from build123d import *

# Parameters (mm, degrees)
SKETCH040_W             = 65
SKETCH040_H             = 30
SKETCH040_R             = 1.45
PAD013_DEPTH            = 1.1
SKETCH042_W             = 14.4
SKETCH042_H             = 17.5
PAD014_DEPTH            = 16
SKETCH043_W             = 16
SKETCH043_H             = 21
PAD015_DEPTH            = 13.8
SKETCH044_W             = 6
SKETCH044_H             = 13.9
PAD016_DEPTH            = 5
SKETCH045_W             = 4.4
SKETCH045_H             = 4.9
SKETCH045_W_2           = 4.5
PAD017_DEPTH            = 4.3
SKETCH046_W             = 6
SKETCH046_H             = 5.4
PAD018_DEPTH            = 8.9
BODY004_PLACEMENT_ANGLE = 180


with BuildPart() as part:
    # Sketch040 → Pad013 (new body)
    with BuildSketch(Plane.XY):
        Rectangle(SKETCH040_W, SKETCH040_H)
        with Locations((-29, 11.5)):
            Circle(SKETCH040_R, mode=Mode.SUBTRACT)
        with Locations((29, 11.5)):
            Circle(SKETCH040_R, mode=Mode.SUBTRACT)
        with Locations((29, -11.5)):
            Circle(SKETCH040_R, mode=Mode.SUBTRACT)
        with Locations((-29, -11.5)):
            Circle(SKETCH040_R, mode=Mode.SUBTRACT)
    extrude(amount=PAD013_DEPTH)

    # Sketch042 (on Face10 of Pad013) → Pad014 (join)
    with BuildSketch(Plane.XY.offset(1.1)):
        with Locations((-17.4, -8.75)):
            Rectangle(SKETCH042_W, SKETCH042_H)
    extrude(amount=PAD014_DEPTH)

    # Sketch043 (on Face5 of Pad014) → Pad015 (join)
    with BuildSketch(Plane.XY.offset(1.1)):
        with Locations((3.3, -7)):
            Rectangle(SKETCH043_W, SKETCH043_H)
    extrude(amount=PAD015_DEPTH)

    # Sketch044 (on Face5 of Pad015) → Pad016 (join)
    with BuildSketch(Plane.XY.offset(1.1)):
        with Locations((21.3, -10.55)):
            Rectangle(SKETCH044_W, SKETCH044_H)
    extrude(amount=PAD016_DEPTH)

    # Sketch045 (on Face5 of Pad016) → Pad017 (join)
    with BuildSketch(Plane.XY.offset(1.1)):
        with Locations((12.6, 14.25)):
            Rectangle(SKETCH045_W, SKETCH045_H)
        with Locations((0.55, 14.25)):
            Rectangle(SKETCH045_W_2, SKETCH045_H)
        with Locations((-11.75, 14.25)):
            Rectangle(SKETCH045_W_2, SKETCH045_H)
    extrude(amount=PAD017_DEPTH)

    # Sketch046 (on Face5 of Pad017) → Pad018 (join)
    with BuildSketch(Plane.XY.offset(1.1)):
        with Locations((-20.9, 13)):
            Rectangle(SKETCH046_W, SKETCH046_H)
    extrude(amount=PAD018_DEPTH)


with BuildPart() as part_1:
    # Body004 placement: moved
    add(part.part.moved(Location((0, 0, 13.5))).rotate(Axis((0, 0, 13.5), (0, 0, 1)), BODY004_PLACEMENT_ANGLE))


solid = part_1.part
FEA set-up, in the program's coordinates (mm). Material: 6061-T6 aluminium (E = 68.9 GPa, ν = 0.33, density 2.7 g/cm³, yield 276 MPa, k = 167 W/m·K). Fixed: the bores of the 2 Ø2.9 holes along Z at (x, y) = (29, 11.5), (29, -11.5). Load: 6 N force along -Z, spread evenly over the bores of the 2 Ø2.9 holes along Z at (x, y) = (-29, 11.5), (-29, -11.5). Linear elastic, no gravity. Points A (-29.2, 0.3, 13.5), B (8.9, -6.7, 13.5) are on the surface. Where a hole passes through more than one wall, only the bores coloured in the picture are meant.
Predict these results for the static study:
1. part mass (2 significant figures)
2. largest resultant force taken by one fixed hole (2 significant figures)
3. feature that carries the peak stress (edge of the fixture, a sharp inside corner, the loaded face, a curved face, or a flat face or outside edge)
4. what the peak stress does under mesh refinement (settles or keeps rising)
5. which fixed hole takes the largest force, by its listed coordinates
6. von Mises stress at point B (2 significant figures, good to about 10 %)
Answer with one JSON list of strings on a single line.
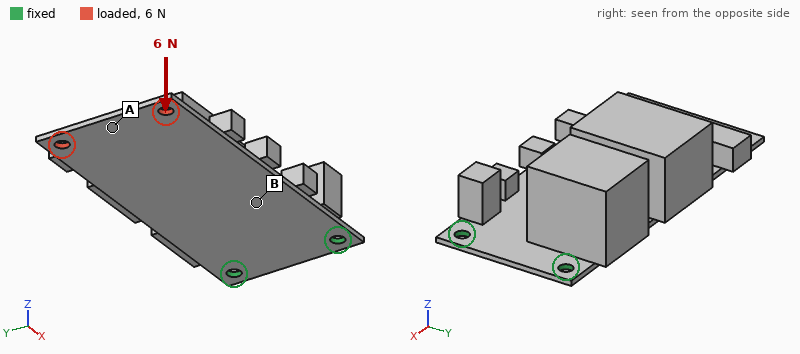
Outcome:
["32 g", "5.6 N", "edge of the fixture", "keeps rising", "(29, -11.5)", "23 MPa"]
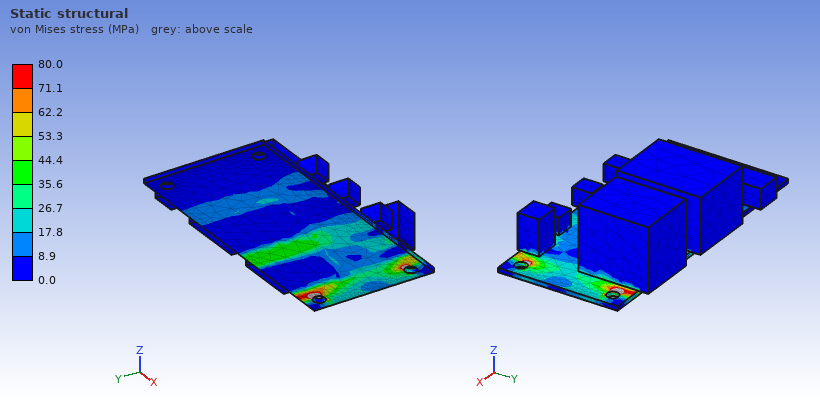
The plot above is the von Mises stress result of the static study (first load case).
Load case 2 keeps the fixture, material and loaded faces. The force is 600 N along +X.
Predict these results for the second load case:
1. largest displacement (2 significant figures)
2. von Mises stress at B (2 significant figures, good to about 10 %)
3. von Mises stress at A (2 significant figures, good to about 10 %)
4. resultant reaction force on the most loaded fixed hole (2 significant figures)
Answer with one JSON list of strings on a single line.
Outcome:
["76 µm", "17 MPa", "8.7 MPa", "310 N"]
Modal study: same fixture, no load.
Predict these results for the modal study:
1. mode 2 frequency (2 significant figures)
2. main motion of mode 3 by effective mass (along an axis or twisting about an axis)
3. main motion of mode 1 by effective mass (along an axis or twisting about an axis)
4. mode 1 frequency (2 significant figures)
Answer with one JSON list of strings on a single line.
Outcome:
["910 Hz", "along Y", "along Z", "190 Hz"]
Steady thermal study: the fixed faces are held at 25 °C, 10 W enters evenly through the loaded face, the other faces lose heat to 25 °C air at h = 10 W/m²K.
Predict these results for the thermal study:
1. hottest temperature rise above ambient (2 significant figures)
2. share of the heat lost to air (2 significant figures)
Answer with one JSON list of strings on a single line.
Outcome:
["77 K", "20 %"]
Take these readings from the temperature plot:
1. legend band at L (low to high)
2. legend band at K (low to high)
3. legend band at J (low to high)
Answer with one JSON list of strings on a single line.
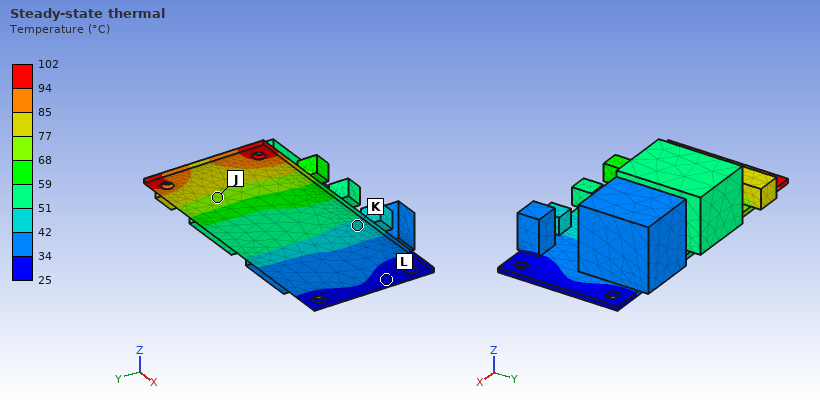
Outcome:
["25 to 34 °C", "42 to 51 °C", "68 to 77 °C"]
